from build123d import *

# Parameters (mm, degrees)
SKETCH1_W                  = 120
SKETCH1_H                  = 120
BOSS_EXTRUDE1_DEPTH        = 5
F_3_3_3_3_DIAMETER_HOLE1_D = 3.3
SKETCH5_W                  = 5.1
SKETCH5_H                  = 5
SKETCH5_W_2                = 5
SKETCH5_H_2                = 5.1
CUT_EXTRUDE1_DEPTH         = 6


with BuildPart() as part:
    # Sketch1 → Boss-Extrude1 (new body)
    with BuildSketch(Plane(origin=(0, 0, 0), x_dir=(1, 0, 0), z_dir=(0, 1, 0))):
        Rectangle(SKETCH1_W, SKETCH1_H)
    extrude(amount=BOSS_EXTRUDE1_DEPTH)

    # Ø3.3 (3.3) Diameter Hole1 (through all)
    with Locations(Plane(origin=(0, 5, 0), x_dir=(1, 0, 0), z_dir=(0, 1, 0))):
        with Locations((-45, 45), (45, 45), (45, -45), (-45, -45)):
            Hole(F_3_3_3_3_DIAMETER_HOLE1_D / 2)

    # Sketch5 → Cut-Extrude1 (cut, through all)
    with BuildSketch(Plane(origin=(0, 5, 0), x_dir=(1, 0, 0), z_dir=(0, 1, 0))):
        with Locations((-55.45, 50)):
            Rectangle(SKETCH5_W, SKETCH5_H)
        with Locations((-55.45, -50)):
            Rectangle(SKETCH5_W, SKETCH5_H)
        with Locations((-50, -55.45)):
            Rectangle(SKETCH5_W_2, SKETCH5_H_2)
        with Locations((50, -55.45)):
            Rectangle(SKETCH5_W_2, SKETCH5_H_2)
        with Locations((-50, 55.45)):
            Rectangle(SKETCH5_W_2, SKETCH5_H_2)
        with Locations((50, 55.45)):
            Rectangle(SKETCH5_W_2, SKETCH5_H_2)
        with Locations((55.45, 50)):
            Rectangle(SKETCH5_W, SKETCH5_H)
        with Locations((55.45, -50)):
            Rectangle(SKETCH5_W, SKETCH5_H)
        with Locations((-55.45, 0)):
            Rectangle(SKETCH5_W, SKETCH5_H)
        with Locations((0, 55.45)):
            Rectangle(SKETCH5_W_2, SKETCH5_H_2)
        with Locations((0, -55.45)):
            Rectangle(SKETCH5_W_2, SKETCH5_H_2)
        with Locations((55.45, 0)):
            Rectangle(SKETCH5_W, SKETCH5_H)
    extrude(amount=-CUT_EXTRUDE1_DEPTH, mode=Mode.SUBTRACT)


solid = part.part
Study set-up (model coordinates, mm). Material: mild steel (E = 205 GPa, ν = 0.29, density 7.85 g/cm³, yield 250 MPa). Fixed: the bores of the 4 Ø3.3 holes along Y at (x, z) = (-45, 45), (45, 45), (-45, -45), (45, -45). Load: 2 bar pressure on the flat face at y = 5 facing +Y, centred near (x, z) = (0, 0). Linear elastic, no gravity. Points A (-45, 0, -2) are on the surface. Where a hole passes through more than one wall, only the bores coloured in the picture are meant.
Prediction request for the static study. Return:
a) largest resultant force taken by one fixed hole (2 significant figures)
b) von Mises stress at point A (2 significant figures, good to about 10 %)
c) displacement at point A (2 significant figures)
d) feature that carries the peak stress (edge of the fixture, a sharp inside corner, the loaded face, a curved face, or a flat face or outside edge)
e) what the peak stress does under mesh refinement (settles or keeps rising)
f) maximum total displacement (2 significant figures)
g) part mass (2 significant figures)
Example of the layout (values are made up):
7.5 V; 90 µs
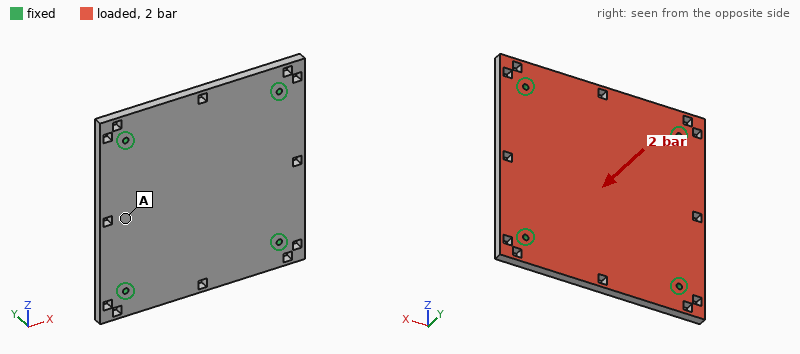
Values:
700 N; 24 MPa; 28 µm; edge of the fixture; keeps rising; 48 µm; 550 g
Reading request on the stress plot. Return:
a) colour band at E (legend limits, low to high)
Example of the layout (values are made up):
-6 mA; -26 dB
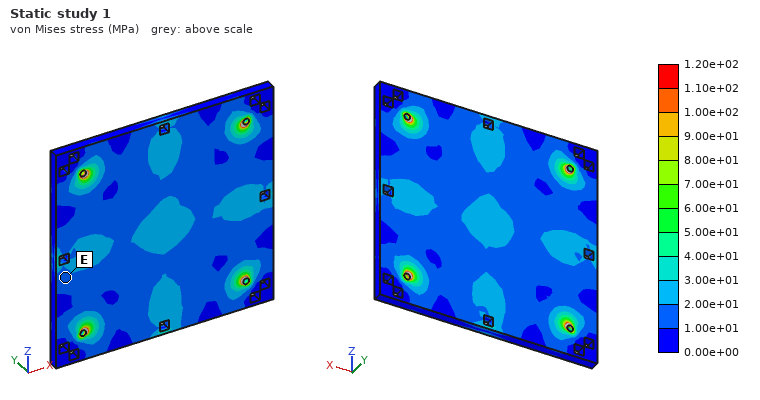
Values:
1.00e+01 to 2.00e+01 MPa
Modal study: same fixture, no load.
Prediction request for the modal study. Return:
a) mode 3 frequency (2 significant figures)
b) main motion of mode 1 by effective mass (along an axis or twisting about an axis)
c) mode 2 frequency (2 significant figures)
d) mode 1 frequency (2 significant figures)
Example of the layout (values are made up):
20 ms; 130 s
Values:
3100 Hz; along Y; 3100 Hz; 2000 Hz
